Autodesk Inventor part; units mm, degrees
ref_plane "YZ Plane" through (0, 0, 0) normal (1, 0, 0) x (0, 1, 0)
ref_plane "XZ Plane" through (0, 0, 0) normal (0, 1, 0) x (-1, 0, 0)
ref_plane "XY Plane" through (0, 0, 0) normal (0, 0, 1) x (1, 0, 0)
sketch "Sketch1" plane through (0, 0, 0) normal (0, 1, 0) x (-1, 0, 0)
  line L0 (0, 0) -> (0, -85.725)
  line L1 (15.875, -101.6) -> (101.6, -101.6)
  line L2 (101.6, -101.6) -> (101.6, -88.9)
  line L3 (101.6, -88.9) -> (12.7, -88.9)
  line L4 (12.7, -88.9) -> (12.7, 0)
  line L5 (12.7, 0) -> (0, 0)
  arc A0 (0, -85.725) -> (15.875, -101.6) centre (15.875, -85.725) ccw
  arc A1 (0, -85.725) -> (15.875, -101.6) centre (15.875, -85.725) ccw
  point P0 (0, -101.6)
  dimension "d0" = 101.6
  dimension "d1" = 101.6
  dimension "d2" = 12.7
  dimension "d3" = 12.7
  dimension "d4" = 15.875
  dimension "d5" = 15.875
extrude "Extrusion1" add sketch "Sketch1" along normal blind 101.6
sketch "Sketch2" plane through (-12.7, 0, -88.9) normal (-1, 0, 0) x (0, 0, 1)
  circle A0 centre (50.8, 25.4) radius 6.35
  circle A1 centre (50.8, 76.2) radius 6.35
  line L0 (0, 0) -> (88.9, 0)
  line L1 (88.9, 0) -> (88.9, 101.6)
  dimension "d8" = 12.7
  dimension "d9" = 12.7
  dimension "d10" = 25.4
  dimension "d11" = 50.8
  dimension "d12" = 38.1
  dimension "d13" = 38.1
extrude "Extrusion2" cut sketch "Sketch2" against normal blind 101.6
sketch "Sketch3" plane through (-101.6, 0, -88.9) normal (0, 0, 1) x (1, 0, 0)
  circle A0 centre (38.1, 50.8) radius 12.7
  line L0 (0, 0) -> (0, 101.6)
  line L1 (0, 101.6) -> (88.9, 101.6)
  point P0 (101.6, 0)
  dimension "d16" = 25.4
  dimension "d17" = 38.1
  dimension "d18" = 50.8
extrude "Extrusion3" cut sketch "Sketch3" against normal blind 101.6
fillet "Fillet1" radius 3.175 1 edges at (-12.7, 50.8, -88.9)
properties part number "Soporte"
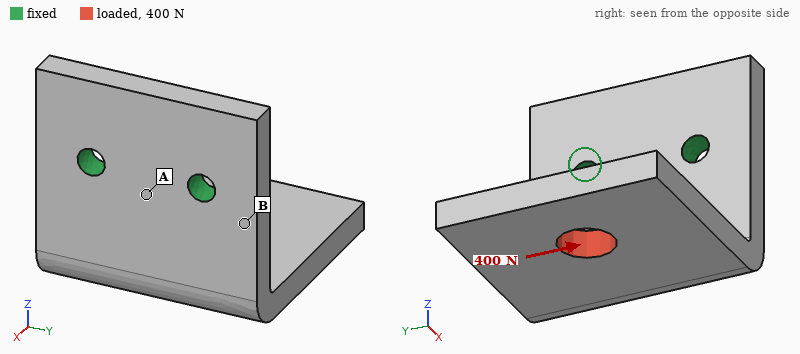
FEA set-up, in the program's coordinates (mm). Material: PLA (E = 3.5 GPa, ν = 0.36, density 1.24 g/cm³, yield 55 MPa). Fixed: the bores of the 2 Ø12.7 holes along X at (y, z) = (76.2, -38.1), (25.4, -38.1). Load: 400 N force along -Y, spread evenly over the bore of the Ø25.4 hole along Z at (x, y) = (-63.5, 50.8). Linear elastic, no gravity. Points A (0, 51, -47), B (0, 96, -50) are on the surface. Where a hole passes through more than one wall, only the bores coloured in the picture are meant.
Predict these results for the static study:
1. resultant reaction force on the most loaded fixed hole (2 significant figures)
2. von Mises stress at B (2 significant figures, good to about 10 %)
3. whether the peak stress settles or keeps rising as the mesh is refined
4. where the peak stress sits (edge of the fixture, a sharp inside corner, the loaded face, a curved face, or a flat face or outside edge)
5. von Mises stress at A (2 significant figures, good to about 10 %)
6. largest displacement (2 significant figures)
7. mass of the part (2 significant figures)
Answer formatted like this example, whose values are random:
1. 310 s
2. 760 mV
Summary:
1. 550 N
2. 4.7 MPa
3. keeps rising
4. edge of the fixture
5. 1.5 MPa
6. 0.84 mm
7. 290 g
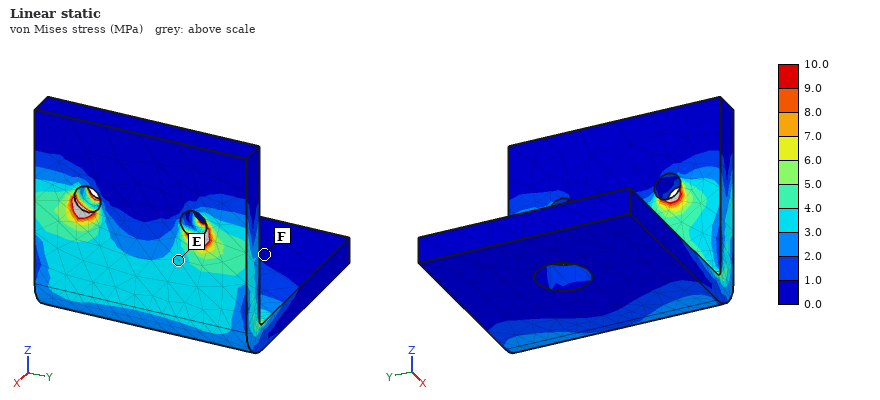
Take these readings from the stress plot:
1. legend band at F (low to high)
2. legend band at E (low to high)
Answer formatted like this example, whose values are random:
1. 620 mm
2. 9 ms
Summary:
1. 0.0 to 1.0 MPa
2. 3.0 to 4.0 MPa
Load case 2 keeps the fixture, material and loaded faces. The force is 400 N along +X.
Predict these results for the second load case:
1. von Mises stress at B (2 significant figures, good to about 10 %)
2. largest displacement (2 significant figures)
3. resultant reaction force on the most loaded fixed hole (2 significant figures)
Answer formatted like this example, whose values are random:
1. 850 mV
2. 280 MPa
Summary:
1. 4.9 MPa
2. 1.0 mm
3. 200 N
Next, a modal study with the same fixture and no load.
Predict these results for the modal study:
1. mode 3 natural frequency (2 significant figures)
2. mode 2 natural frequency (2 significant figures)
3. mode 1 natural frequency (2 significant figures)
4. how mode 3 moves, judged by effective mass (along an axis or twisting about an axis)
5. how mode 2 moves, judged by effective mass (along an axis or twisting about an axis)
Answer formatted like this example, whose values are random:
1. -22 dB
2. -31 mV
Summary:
1. 630 Hz
2. 360 Hz
3. 210 Hz
4. along X
5. along Y
